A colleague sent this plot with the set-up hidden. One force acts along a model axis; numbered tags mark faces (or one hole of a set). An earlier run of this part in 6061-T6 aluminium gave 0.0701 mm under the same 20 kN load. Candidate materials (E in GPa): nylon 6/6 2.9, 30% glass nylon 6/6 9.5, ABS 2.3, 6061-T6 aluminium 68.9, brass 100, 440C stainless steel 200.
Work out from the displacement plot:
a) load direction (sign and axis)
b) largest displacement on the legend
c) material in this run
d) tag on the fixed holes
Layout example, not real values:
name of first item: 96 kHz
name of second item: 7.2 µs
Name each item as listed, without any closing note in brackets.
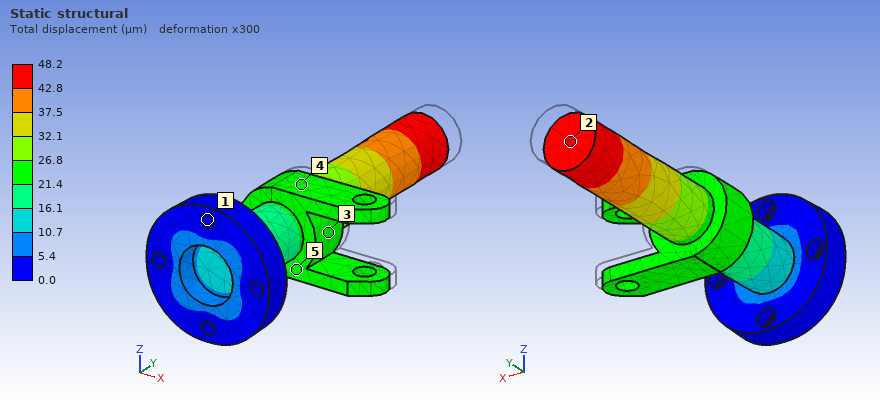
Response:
load direction: -Y
largest displacement on the legend: 48.2 µm
material in this run: brass
tag on the fixed holes: 1
